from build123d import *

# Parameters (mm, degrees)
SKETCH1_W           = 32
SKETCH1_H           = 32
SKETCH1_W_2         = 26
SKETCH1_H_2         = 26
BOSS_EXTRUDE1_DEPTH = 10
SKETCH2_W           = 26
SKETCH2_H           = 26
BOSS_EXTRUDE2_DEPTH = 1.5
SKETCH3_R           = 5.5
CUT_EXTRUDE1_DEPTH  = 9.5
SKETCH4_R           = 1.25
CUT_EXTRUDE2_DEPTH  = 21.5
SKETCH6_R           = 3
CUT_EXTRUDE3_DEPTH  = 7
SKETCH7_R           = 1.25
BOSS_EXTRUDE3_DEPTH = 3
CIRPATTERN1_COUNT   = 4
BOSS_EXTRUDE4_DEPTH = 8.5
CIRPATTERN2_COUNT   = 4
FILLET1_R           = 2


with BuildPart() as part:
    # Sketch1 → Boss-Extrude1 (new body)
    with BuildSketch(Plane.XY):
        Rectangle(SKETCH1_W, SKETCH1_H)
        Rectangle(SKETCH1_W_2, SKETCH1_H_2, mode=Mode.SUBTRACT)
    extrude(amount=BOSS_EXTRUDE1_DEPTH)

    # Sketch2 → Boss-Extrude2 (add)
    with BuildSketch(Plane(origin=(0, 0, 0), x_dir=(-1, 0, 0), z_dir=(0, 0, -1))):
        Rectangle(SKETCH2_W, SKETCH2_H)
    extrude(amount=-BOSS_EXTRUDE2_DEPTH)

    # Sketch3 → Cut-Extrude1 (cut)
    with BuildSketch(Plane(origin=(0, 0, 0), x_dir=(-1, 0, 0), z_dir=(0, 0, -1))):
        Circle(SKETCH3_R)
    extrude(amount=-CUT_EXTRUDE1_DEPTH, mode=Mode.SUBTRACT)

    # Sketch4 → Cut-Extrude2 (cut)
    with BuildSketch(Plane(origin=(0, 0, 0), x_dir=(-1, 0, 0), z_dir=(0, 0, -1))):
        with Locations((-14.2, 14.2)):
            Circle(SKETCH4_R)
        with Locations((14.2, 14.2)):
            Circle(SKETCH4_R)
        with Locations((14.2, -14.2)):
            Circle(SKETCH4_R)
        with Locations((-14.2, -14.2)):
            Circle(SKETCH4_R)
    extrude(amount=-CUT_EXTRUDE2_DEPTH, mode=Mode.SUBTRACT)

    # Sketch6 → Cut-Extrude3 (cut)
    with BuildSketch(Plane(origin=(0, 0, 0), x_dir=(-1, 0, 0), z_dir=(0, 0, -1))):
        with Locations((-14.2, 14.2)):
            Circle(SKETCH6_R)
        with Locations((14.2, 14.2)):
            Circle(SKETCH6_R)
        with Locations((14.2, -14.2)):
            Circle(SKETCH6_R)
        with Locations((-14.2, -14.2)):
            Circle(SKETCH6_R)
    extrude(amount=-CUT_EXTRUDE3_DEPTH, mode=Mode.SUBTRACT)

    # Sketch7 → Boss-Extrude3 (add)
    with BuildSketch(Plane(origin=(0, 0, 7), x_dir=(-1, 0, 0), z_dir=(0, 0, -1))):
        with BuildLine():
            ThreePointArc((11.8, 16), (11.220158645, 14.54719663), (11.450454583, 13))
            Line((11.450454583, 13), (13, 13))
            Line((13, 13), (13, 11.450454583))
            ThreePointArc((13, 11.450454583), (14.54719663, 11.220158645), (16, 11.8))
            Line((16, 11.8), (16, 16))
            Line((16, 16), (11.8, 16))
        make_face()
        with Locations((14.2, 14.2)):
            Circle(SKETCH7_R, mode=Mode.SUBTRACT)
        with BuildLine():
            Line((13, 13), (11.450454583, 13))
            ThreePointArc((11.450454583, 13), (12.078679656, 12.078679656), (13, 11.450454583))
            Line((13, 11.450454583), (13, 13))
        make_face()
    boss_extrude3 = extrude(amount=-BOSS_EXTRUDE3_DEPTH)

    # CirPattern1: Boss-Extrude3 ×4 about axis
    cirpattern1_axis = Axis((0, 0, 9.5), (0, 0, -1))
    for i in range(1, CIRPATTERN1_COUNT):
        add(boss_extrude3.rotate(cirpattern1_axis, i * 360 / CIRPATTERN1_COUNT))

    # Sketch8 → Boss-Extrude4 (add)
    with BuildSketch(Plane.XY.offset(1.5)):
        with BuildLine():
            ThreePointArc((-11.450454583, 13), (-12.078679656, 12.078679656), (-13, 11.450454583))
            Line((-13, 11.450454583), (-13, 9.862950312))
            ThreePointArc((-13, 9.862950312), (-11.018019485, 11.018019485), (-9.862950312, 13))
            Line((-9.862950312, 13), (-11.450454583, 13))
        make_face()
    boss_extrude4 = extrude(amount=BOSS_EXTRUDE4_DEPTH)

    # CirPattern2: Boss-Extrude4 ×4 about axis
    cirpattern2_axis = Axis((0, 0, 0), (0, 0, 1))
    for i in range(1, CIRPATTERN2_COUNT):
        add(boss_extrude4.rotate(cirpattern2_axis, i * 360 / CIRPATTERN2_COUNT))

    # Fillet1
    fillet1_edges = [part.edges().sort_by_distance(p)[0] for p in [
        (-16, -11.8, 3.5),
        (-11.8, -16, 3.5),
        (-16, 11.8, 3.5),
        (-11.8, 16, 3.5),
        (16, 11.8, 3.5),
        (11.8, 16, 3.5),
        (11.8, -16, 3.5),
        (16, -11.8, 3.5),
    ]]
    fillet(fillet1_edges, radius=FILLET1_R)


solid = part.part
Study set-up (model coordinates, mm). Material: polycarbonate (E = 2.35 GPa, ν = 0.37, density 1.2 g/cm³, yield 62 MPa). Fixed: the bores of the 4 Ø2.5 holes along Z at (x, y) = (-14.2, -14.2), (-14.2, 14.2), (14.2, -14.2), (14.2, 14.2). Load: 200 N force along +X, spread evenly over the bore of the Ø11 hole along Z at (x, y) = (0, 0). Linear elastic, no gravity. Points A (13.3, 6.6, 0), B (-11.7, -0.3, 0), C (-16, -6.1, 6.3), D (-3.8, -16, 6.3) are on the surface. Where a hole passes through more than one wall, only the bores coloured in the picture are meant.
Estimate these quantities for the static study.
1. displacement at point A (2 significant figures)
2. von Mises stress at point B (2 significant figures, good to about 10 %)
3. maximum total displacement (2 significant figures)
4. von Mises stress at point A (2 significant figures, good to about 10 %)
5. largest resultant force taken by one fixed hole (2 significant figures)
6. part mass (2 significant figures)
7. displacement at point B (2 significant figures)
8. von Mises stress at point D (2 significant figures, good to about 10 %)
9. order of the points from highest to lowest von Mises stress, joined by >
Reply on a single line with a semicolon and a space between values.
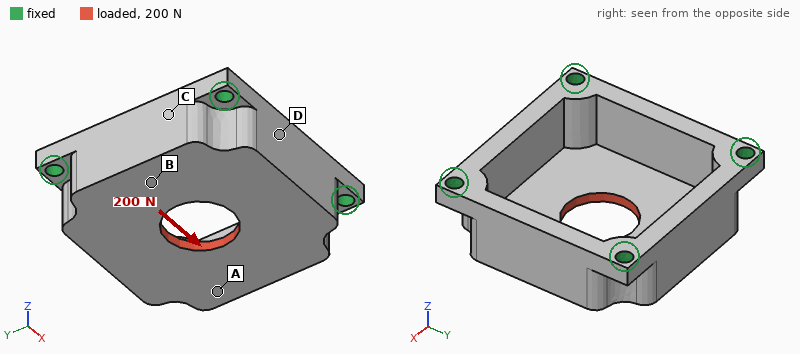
46 µm; 2.6 MPa; 64 µm; 3.7 MPa; 58 N; 4.7 g; 56 µm; 1.5 MPa; A > B > D > C
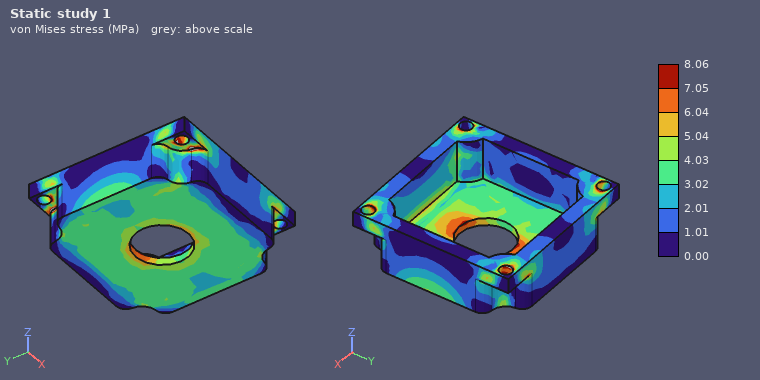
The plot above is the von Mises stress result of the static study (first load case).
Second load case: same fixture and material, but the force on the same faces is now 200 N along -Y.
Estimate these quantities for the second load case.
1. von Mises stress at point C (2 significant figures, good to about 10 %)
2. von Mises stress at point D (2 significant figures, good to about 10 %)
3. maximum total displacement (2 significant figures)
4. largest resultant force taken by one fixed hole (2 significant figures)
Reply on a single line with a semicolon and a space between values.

2.0 MPa; 0.99 MPa; 64 µm; 58 N
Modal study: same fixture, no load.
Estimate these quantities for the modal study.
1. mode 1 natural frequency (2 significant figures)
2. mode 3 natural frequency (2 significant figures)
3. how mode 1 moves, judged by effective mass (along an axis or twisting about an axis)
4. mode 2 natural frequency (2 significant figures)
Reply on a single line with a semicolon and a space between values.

5000 Hz; 6800 Hz; along Z; 6700 Hz
